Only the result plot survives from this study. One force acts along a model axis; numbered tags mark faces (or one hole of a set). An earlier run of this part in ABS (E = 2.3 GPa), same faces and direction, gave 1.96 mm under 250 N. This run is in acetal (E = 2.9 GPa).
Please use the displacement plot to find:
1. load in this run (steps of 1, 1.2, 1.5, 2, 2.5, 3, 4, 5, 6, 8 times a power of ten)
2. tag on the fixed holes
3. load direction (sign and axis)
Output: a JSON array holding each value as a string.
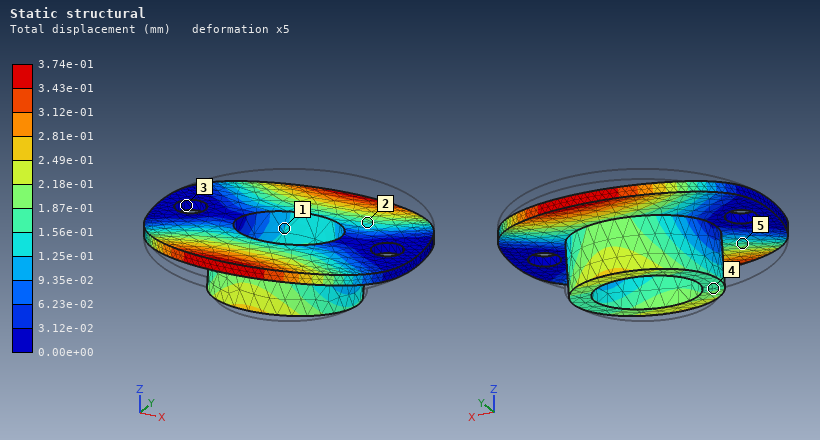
["60 N", "3", "-Y"]
